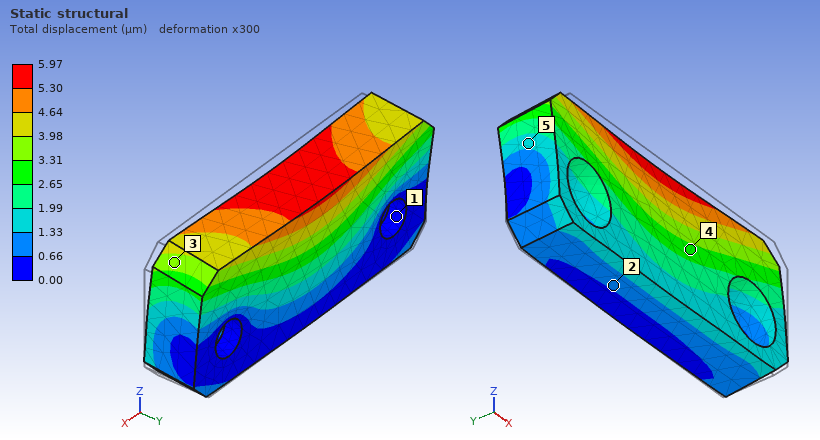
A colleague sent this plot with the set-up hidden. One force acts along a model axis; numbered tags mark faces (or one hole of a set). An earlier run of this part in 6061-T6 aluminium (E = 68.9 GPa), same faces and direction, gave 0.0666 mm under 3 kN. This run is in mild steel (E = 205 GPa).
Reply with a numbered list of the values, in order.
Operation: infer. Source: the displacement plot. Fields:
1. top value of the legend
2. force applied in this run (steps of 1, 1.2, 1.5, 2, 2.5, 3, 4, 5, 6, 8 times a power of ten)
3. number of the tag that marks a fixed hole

1. 5.97 µm
2. 800 N
3. 1
